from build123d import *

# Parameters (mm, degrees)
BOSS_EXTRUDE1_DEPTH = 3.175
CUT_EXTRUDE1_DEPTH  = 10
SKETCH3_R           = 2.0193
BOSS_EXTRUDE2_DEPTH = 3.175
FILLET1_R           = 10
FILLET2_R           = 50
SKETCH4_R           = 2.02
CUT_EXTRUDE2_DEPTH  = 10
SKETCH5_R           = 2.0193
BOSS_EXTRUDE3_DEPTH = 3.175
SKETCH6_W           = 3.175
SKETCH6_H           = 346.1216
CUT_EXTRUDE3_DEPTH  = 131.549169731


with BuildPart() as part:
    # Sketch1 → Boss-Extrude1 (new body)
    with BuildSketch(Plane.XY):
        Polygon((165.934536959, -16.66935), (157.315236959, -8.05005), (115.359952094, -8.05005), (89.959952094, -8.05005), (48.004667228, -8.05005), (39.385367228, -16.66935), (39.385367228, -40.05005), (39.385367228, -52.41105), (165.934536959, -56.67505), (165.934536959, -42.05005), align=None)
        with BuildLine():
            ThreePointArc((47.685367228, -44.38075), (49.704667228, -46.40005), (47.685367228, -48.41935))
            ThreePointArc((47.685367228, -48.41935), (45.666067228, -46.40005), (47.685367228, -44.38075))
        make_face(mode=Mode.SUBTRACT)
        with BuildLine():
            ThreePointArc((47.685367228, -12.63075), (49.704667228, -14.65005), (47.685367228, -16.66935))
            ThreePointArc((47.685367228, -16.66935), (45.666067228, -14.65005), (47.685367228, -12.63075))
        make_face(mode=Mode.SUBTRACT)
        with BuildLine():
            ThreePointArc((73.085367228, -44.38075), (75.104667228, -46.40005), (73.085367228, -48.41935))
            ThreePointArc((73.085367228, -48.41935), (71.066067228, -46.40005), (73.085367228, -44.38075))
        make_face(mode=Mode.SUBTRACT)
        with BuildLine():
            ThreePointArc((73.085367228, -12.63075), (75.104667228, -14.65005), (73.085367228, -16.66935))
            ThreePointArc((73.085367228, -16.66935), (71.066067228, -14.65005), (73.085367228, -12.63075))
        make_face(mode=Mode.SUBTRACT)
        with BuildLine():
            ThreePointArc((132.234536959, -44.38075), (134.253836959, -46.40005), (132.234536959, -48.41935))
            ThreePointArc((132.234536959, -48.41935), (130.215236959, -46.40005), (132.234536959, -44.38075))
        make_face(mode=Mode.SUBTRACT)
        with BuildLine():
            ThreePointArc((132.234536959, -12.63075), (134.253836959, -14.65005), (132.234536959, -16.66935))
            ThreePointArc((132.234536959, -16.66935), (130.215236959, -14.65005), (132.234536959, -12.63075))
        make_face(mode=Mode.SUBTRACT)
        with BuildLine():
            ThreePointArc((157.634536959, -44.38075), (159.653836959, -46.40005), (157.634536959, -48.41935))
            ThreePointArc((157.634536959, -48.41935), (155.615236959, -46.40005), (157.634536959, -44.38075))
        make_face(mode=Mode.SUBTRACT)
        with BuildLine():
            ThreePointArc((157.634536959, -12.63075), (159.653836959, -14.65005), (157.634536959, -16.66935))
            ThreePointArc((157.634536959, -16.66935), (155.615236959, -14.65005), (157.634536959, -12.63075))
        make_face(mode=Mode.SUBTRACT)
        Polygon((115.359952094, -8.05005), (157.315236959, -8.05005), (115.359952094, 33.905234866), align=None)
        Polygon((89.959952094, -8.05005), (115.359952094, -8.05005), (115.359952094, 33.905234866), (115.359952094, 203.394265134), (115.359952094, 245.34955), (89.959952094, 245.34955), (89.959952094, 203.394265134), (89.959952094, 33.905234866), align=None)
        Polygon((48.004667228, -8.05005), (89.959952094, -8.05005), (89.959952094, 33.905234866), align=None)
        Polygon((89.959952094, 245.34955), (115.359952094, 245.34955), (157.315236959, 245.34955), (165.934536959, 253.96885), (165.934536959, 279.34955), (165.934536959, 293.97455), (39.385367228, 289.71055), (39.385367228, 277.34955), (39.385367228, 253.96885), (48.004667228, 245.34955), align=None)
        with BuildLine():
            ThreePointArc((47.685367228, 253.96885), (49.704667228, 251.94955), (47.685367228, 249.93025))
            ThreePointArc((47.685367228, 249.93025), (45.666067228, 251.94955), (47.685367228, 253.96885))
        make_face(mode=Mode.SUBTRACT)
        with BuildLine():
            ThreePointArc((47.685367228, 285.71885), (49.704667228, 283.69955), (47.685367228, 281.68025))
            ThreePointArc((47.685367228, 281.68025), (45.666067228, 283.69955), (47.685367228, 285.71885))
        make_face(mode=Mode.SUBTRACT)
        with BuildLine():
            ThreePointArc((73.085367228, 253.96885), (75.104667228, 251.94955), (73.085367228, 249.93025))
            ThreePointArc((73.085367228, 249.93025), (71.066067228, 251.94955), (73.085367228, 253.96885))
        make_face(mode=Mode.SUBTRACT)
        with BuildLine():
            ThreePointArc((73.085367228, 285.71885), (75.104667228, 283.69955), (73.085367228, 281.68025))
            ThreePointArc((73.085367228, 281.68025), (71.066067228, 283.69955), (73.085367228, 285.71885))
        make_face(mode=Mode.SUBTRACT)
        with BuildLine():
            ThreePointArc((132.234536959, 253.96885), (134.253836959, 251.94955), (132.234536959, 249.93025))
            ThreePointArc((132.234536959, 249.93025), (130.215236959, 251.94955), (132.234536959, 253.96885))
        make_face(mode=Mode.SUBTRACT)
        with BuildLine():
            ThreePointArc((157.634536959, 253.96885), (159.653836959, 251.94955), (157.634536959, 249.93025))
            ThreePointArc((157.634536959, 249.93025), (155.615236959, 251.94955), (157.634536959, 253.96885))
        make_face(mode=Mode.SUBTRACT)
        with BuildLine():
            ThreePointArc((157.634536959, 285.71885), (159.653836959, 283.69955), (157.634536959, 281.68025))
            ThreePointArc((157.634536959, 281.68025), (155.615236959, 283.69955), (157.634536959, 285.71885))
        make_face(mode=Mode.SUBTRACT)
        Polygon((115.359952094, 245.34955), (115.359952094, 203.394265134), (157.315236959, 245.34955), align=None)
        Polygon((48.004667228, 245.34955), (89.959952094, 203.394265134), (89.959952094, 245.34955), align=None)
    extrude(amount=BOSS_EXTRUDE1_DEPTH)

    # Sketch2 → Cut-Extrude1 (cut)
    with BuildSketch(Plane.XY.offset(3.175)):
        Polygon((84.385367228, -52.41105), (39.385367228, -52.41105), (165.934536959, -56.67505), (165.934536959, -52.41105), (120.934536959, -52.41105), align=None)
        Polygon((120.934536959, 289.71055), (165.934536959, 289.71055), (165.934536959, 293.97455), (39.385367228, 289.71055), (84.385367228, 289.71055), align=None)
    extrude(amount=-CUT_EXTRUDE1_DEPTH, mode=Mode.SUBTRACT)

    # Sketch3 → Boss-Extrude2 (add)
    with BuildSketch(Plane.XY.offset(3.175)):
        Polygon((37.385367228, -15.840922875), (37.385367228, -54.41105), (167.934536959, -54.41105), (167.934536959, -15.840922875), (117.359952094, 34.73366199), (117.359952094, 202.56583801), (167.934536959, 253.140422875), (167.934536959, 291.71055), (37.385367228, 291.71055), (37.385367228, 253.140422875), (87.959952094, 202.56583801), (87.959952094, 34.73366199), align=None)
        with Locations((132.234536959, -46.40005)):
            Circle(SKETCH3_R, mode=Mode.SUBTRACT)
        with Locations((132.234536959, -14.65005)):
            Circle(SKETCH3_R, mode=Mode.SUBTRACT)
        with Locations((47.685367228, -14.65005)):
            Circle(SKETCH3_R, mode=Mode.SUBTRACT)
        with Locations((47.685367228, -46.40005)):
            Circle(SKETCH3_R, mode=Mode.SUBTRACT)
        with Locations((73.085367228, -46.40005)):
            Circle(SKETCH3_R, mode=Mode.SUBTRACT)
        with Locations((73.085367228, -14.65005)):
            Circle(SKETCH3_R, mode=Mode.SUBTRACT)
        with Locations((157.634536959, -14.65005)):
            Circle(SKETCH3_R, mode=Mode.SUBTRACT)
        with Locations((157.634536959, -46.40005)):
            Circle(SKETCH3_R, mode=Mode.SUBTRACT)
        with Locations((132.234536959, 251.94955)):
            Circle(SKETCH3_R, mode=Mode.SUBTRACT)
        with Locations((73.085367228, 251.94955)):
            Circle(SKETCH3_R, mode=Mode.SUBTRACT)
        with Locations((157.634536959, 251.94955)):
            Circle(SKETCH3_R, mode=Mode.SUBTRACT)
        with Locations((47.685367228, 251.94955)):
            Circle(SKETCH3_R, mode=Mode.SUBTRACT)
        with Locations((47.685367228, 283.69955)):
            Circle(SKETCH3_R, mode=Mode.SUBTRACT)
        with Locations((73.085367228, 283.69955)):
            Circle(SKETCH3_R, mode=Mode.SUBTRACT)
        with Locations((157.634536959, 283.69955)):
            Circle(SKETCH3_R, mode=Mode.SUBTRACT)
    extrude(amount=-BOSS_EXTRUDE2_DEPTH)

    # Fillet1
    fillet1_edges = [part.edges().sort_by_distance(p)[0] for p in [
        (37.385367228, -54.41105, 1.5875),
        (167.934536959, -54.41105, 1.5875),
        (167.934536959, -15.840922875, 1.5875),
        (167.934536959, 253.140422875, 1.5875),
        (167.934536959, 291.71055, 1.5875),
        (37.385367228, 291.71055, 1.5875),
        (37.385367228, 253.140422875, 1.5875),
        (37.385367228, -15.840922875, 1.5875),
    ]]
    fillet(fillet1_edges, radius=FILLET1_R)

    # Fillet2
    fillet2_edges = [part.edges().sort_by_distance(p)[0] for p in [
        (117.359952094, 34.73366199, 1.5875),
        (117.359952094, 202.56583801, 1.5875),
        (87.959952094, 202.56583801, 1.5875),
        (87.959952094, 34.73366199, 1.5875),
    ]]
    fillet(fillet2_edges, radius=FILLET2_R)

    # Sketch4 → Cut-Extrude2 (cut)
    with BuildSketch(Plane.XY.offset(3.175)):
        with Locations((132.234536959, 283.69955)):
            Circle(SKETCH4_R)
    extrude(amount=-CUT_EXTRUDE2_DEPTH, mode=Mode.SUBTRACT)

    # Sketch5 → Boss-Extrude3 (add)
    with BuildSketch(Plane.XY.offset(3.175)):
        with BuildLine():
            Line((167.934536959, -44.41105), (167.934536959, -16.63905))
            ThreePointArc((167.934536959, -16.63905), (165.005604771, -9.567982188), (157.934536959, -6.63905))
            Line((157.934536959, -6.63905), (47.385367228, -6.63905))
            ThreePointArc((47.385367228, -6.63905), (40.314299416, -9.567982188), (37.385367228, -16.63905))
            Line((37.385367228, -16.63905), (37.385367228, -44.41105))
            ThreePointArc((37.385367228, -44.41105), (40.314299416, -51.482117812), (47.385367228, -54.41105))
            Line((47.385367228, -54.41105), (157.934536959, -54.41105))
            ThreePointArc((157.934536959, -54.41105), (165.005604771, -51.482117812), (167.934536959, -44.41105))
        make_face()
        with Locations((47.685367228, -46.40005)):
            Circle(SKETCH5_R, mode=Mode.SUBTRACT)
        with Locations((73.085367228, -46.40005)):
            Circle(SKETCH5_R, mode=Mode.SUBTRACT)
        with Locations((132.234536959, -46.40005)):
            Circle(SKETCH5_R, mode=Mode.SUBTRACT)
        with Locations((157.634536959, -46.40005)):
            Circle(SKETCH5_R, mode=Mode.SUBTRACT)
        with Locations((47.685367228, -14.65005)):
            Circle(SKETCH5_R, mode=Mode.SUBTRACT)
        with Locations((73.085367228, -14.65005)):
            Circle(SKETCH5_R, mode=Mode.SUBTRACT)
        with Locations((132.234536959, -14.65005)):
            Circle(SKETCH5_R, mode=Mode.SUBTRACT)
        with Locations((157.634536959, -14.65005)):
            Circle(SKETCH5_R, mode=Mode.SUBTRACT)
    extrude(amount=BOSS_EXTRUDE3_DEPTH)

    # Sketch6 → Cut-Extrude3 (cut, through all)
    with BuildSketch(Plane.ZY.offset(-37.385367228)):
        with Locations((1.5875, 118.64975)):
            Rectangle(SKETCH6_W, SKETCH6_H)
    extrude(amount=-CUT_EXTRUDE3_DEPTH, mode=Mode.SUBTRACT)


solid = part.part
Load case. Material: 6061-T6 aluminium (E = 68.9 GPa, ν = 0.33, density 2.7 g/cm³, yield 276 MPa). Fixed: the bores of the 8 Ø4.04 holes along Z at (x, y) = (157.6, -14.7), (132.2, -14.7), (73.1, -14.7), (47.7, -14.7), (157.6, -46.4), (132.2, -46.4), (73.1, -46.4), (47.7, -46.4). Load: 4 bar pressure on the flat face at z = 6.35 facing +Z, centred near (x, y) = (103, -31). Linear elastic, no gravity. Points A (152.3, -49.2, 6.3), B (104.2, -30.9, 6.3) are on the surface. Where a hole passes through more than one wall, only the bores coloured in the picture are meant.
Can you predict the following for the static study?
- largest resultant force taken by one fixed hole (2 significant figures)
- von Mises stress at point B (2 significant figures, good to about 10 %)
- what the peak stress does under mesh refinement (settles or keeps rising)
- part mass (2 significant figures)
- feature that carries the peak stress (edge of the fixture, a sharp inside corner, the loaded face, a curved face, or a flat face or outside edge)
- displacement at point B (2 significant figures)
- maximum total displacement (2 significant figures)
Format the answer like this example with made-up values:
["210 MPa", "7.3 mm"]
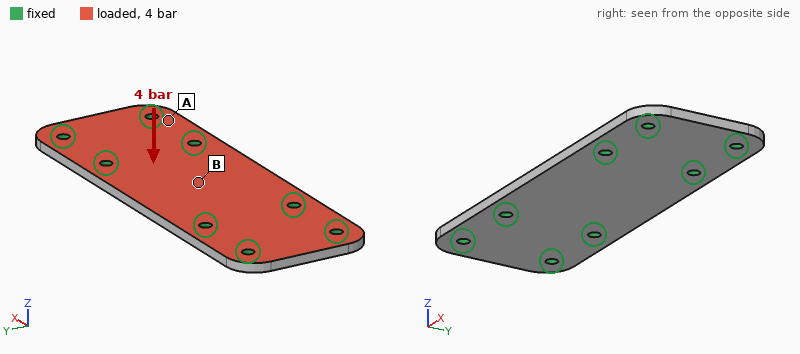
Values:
["420 N", "29 MPa", "keeps rising", "52 g", "edge of the fixture", "72 µm", "73 µm"]
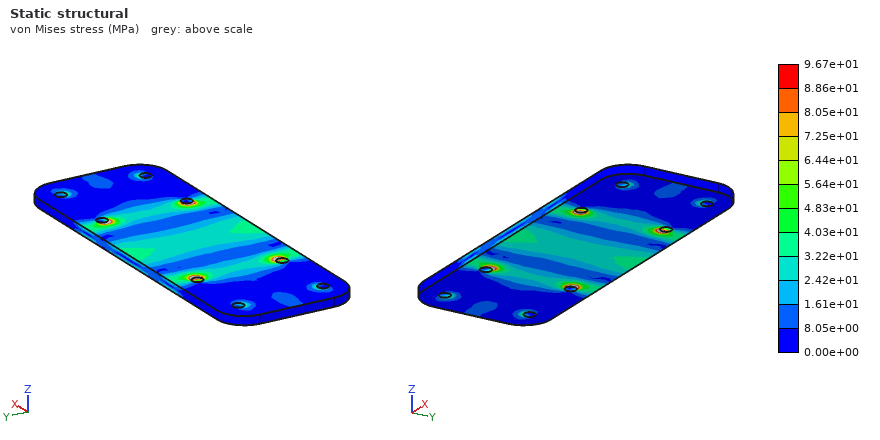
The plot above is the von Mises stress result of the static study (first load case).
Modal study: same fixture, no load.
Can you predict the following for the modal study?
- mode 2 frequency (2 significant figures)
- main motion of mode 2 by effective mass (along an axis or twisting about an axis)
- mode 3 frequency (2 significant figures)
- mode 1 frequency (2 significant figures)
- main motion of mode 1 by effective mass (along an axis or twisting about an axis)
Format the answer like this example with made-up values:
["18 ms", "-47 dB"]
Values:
["6100 Hz", "twisting about X", "11 kHz", "4600 Hz", "along Z"]
